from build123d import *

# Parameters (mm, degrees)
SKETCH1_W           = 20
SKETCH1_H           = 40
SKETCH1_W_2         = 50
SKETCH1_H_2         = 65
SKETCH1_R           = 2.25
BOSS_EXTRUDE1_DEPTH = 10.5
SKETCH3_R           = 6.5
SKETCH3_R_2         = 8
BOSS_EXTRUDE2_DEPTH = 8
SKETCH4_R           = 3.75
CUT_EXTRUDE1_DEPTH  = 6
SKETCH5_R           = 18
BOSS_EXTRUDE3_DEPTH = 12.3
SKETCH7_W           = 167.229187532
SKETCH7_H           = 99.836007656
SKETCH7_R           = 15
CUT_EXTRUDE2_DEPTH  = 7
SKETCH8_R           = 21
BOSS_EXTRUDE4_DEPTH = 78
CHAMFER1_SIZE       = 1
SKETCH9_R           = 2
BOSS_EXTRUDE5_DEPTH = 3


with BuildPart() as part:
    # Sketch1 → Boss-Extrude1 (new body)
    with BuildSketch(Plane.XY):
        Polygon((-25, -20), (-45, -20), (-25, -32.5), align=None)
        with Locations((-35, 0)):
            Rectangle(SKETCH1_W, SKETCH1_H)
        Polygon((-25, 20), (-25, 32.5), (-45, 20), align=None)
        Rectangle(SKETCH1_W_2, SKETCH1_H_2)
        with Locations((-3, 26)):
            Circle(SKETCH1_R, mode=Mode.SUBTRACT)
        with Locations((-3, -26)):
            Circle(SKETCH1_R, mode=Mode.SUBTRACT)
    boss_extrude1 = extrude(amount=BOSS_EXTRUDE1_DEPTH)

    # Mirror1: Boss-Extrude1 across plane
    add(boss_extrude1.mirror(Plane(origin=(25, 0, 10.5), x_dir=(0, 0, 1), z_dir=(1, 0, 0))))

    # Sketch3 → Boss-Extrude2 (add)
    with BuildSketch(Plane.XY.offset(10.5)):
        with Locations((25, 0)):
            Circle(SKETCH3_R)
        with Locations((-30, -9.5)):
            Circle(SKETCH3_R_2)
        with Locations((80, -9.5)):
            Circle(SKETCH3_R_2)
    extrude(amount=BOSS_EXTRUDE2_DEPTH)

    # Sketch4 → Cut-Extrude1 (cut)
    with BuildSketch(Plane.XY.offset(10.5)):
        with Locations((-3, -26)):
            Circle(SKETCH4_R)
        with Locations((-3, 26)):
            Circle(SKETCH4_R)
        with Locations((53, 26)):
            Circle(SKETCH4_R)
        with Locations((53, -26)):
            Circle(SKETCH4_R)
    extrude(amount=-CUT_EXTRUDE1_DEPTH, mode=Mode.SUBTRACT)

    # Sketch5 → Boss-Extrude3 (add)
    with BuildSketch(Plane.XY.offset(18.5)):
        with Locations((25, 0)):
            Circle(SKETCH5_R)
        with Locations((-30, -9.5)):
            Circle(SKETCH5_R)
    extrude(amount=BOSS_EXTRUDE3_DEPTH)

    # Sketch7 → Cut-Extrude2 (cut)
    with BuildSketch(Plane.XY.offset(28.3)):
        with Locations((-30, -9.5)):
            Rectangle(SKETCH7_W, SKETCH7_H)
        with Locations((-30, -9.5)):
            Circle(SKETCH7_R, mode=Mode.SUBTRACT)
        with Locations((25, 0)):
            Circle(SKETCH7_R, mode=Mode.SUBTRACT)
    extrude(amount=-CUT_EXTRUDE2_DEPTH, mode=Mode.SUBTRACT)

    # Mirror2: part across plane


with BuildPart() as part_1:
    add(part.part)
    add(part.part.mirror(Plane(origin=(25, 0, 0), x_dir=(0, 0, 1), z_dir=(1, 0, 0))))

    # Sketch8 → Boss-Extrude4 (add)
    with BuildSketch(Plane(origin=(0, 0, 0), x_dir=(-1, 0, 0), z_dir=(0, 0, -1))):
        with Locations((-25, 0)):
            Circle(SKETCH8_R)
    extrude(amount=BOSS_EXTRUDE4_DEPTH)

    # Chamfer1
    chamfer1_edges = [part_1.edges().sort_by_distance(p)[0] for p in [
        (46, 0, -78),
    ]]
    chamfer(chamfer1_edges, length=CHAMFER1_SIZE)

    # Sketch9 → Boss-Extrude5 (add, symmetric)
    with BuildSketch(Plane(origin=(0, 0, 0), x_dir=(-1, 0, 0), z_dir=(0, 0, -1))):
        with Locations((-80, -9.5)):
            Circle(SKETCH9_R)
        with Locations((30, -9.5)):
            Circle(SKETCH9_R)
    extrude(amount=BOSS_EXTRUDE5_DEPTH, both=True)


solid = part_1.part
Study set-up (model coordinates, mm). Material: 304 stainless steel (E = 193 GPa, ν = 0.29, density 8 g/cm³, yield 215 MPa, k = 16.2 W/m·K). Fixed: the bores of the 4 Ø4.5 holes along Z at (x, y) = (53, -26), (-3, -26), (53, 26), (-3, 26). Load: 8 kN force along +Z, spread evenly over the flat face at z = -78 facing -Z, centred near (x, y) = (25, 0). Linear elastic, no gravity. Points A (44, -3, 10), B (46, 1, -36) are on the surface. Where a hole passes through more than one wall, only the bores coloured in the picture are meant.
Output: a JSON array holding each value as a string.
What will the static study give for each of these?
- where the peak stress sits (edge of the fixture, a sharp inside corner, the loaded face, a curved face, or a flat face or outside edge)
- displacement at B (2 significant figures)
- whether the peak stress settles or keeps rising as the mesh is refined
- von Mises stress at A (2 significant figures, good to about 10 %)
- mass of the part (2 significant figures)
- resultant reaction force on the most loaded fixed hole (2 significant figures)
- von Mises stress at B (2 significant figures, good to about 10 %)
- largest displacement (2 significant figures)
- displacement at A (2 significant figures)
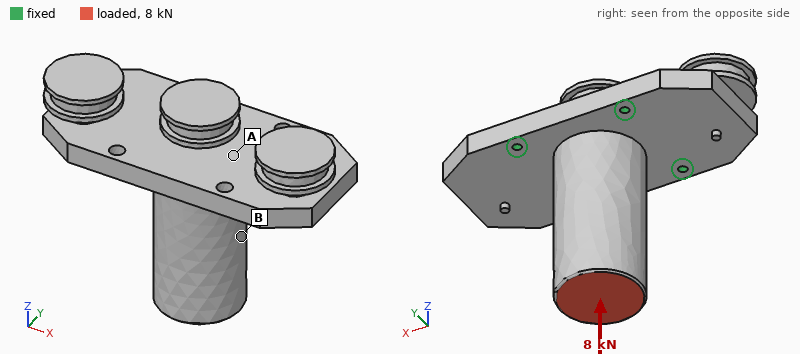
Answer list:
["edge of the fixture", "10 µm", "keeps rising", "25 MPa", "1.9 kg", "2.3 kN", "5.7 MPa", "12 µm", "8.6 µm"]
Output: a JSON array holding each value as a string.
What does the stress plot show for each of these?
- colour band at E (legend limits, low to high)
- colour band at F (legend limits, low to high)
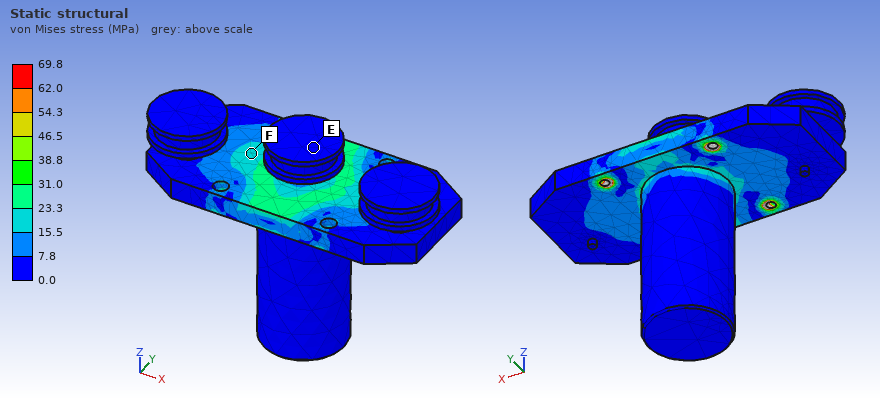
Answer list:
["0.0 to 7.8 MPa", "15.5 to 23.3 MPa"]
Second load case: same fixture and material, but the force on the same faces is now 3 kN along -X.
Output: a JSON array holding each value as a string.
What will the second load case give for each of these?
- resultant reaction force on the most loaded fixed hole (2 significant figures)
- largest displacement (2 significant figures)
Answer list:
["2.5 kN", "56 µm"]
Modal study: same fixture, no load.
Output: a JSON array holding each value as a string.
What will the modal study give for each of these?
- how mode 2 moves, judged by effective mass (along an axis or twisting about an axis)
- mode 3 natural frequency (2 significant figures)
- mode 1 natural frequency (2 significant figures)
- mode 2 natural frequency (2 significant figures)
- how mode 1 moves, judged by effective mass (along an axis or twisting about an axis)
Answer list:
["along X", "2300 Hz", "1900 Hz", "2100 Hz", "along Y"]
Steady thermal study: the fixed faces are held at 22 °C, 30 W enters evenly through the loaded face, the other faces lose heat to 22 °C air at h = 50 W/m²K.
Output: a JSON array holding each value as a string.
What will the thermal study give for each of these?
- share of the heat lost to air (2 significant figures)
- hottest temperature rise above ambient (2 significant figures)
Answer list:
["82 %", "76 K"]
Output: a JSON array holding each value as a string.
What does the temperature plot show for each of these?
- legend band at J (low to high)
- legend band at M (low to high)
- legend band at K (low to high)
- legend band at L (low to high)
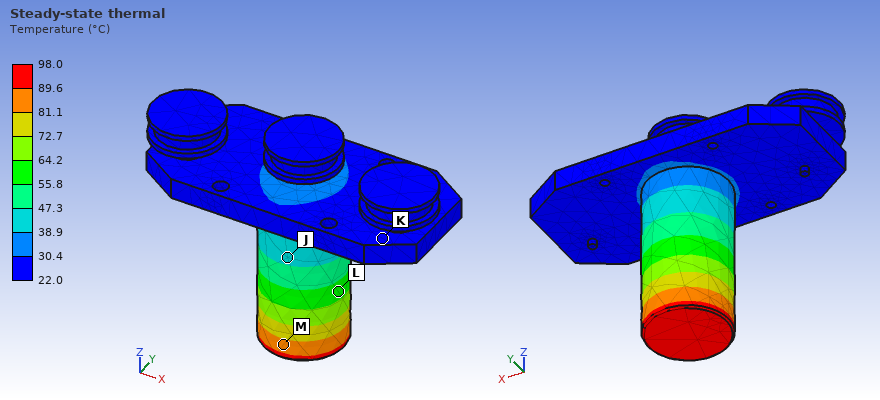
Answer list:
["38.9 to 47.3 °C", "81.1 to 89.6 °C", "22.0 to 30.4 °C", "55.8 to 64.2 °C"]
